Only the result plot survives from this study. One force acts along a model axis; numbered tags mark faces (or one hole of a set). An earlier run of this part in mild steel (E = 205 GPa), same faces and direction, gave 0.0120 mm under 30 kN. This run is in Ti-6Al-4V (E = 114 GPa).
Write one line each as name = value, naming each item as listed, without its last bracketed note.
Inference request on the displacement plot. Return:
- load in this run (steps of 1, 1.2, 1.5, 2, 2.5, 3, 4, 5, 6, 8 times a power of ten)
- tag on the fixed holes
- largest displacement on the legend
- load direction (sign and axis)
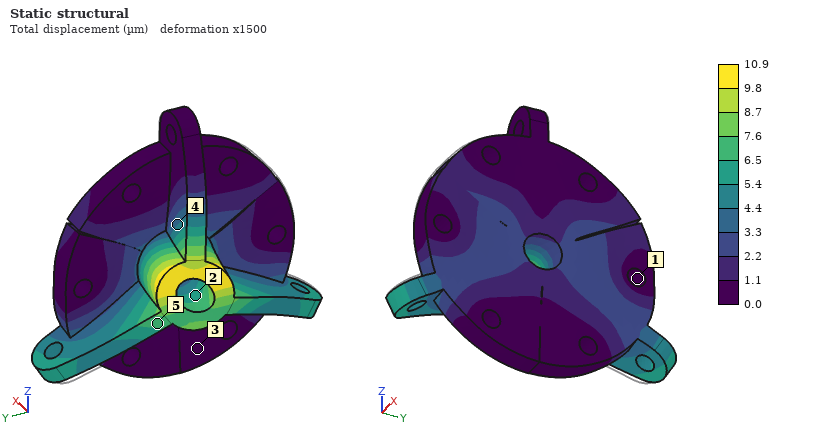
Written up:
load in this run = 15 kN
tag on the fixed holes = 1
largest displacement on the legend = 10.9 µm
load direction = +Y
